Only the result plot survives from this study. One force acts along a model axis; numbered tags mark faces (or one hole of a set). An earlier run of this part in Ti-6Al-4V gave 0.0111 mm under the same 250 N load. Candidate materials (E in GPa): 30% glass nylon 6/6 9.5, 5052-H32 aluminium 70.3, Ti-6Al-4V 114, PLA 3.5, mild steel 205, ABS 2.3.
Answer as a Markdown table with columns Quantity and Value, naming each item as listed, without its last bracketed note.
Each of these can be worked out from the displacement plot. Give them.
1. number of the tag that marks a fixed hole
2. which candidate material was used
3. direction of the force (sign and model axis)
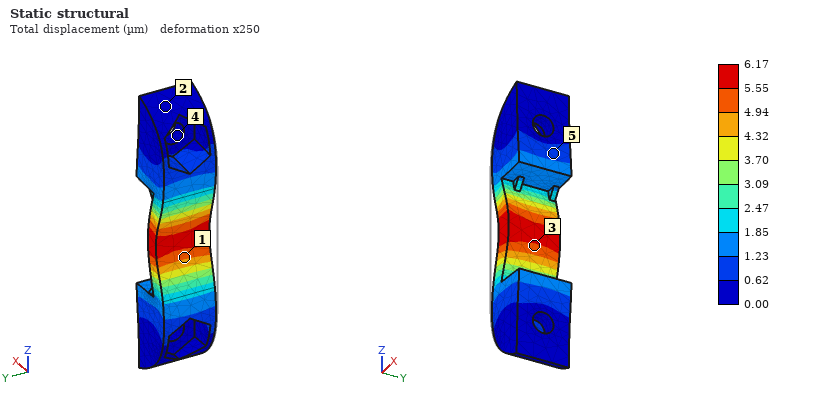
| Quantity | Value |
|---|---|
| number of the tag that marks a fixed hole | 4 |
| which candidate material was used | mild steel |
| direction of the force | +X |
